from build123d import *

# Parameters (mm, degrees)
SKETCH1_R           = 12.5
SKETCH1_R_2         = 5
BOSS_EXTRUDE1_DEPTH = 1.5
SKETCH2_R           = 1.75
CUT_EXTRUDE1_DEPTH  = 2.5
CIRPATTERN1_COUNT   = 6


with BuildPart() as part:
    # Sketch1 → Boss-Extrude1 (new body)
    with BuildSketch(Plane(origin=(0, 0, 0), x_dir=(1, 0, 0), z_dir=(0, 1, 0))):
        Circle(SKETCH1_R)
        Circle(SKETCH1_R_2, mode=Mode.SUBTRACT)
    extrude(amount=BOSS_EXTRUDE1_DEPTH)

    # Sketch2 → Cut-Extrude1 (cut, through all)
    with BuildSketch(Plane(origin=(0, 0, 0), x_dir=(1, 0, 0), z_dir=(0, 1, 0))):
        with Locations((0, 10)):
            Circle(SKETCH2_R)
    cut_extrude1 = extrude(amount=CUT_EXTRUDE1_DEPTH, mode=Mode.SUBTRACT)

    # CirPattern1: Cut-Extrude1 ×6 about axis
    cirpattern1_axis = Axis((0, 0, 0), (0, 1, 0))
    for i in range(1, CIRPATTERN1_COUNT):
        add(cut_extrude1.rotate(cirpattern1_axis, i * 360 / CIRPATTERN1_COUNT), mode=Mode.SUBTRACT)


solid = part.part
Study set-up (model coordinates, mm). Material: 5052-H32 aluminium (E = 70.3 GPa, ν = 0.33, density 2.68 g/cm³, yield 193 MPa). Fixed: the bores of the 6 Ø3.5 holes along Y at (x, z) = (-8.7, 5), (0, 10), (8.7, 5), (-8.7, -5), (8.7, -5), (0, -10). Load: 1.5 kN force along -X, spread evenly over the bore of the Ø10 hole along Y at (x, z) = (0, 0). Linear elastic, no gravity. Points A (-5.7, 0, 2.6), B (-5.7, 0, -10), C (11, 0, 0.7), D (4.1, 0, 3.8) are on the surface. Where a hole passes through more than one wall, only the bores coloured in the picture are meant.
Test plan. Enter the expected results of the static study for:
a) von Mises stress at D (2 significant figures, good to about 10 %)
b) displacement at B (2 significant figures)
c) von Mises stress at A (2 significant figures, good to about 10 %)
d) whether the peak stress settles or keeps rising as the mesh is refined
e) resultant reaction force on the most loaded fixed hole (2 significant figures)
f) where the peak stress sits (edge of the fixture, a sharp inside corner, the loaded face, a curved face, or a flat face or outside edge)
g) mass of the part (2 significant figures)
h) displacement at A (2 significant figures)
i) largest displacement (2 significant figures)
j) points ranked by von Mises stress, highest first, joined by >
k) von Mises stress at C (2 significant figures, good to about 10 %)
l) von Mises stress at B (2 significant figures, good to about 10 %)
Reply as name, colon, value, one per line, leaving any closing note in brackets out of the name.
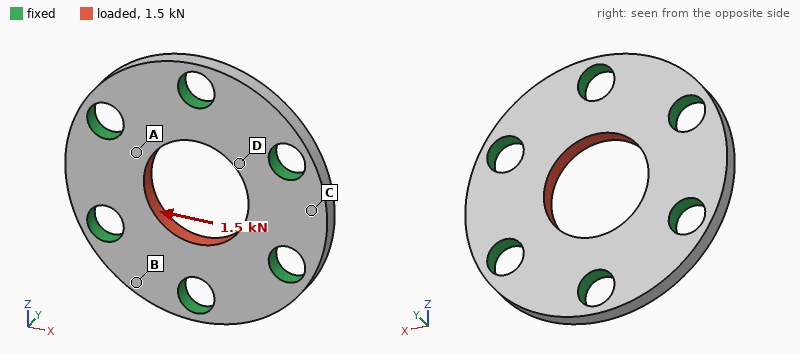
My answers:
von Mises stress at D: 43 MPa
displacement at B: 0.53 µm
von Mises stress at A: 33 MPa
whether the peak stress settles or keeps rising as the mesh is refined: keeps rising
resultant reaction force on the most loaded fixed hole: 320 N
where the peak stress sits: edge of the fixture
mass of the part: 1.4 g
displacement at A: 1.4 µm
largest displacement: 2.7 µm
points ranked by von Mises stress, highest first, joined by >: D > A > C > B
von Mises stress at C: 9.2 MPa
von Mises stress at B: 4.9 MPa
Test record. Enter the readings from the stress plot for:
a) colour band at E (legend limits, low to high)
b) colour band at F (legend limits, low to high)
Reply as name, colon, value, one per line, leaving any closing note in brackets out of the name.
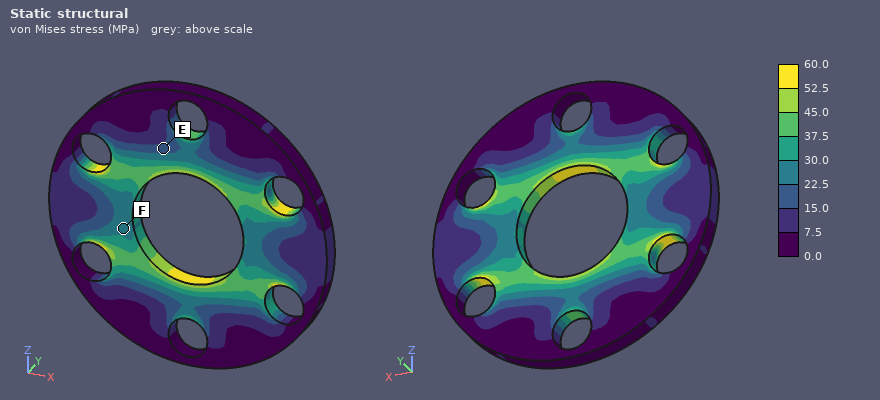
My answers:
colour band at E: 15.0 to 22.5 MPa
colour band at F: 22.5 to 30.0 MPa
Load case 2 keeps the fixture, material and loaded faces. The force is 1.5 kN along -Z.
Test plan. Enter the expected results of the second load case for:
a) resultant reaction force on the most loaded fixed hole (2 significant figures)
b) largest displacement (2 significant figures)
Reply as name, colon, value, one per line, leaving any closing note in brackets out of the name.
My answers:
resultant reaction force on the most loaded fixed hole: 360 N
largest displacement: 2.6 µm
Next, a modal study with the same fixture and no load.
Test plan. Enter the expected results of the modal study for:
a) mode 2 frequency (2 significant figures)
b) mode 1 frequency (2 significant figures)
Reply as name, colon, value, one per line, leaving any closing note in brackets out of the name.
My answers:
mode 2 frequency: 90 kHz
mode 1 frequency: 82 kHz
